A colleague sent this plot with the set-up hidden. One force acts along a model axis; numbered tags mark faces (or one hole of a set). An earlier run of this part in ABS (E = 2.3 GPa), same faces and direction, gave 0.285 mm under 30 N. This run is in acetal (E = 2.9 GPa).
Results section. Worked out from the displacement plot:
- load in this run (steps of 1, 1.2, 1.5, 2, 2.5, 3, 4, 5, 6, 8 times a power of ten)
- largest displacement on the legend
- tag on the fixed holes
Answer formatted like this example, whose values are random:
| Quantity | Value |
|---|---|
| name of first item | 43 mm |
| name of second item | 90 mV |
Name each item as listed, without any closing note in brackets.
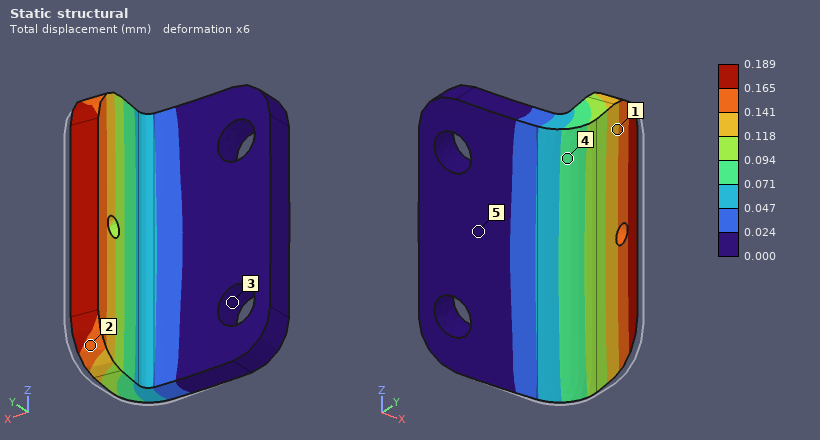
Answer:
| Quantity | Value |
|---|---|
| load in this run | 25 N |
| largest displacement on the legend | 0.189 mm |
| tag on the fixed holes | 3 |
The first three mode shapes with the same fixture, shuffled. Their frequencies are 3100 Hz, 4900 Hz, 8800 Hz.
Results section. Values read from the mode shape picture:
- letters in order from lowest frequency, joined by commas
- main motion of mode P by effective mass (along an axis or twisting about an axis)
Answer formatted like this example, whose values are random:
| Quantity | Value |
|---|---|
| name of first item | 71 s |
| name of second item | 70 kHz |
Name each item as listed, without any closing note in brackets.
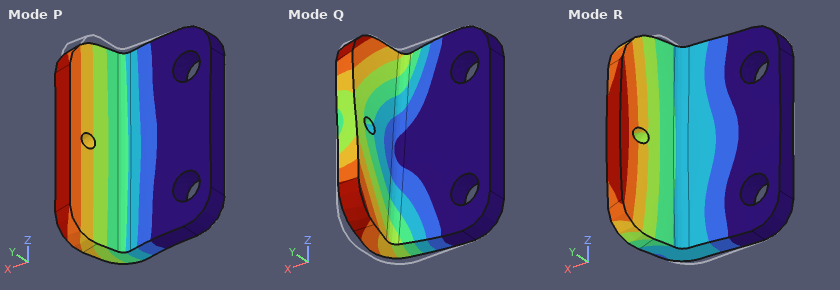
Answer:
| Quantity | Value |
|---|---|
| letters in order from lowest frequency, joined by commas | P, Q, R |
| main motion of mode P by effective mass | along Y |
